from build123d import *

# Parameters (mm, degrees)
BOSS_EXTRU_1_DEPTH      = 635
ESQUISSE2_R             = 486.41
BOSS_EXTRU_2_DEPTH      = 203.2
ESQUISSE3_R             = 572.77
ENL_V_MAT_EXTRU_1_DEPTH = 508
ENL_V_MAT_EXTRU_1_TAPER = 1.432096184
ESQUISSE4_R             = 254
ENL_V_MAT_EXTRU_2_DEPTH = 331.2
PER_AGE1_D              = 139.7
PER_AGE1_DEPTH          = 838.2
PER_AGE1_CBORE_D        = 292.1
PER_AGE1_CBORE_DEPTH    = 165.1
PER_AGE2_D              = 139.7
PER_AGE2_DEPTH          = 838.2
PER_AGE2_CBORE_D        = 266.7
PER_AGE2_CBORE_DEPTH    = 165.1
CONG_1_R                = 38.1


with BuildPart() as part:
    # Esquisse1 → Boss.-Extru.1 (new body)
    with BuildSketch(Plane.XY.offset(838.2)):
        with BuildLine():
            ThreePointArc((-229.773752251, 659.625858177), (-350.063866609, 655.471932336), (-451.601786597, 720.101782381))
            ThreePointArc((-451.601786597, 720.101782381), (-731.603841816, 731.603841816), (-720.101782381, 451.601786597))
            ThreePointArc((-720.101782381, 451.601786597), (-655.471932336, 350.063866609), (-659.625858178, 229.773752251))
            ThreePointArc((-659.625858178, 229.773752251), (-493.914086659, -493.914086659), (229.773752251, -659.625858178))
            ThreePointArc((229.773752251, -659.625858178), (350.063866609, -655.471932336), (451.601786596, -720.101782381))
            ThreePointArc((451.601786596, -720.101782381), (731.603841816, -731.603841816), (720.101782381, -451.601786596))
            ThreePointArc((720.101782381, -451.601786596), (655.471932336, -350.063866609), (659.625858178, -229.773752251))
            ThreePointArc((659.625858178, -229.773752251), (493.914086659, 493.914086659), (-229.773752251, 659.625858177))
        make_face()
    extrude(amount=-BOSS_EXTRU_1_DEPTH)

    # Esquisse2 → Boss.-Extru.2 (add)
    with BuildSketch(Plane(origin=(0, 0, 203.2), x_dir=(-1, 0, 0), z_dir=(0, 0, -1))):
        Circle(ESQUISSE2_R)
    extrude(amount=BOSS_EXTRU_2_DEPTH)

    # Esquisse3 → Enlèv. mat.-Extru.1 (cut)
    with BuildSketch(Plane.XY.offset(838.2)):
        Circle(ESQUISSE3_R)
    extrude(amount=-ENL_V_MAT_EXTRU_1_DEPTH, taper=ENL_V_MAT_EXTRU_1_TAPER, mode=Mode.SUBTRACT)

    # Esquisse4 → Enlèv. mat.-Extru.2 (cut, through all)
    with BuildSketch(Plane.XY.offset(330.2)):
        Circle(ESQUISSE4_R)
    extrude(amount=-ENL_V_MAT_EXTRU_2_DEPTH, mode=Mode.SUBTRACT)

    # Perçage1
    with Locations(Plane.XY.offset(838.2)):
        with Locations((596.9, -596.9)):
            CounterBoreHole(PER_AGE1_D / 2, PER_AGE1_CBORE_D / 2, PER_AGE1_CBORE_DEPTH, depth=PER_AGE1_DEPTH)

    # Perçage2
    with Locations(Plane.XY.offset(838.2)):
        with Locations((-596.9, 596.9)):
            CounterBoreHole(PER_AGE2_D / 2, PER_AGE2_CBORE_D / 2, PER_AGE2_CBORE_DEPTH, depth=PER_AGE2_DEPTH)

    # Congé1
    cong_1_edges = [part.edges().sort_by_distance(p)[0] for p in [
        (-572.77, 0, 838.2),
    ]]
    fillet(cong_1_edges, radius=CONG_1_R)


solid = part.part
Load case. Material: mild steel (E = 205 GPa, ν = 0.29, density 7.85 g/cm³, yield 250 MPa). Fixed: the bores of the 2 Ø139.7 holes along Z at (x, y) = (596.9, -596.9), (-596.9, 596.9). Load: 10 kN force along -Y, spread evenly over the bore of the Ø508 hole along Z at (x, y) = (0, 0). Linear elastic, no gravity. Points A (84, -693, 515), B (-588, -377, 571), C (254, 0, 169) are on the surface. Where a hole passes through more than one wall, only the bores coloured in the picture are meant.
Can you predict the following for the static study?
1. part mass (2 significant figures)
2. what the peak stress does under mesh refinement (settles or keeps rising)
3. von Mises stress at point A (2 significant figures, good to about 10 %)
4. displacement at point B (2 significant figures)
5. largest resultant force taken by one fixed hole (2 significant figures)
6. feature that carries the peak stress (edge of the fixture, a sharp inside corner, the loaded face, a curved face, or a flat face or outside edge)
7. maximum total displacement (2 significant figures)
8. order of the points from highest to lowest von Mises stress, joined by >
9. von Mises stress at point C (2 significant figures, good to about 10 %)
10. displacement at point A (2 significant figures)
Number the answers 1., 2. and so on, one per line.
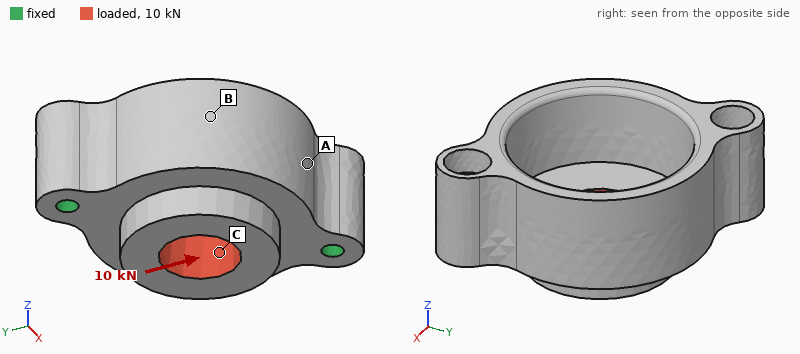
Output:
1. 5200 kg
2. keeps rising
3. 0.028 MPa
4. 0.40 µm
5. 5.1 kN
6. edge of the fixture
7. 0.54 µm
8. C > A > B
9. 0.050 MPa
10. 0.26 µm
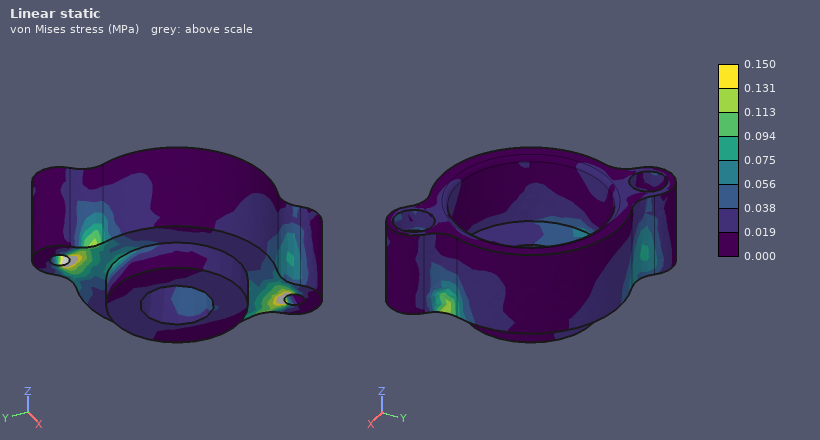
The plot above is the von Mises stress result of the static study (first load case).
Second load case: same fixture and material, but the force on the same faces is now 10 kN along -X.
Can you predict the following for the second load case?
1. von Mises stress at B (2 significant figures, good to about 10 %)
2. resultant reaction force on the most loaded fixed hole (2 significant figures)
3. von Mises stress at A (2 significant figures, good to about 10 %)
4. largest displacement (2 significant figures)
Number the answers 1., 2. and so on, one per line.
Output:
1. 0.013 MPa
2. 5.1 kN
3. 0.025 MPa
4. 0.54 µm
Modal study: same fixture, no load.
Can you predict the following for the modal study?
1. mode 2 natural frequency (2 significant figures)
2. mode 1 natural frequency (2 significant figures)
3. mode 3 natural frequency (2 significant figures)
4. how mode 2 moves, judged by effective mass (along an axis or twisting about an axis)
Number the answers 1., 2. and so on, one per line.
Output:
1. 420 Hz
2. 310 Hz
3. 510 Hz
4. along Z
